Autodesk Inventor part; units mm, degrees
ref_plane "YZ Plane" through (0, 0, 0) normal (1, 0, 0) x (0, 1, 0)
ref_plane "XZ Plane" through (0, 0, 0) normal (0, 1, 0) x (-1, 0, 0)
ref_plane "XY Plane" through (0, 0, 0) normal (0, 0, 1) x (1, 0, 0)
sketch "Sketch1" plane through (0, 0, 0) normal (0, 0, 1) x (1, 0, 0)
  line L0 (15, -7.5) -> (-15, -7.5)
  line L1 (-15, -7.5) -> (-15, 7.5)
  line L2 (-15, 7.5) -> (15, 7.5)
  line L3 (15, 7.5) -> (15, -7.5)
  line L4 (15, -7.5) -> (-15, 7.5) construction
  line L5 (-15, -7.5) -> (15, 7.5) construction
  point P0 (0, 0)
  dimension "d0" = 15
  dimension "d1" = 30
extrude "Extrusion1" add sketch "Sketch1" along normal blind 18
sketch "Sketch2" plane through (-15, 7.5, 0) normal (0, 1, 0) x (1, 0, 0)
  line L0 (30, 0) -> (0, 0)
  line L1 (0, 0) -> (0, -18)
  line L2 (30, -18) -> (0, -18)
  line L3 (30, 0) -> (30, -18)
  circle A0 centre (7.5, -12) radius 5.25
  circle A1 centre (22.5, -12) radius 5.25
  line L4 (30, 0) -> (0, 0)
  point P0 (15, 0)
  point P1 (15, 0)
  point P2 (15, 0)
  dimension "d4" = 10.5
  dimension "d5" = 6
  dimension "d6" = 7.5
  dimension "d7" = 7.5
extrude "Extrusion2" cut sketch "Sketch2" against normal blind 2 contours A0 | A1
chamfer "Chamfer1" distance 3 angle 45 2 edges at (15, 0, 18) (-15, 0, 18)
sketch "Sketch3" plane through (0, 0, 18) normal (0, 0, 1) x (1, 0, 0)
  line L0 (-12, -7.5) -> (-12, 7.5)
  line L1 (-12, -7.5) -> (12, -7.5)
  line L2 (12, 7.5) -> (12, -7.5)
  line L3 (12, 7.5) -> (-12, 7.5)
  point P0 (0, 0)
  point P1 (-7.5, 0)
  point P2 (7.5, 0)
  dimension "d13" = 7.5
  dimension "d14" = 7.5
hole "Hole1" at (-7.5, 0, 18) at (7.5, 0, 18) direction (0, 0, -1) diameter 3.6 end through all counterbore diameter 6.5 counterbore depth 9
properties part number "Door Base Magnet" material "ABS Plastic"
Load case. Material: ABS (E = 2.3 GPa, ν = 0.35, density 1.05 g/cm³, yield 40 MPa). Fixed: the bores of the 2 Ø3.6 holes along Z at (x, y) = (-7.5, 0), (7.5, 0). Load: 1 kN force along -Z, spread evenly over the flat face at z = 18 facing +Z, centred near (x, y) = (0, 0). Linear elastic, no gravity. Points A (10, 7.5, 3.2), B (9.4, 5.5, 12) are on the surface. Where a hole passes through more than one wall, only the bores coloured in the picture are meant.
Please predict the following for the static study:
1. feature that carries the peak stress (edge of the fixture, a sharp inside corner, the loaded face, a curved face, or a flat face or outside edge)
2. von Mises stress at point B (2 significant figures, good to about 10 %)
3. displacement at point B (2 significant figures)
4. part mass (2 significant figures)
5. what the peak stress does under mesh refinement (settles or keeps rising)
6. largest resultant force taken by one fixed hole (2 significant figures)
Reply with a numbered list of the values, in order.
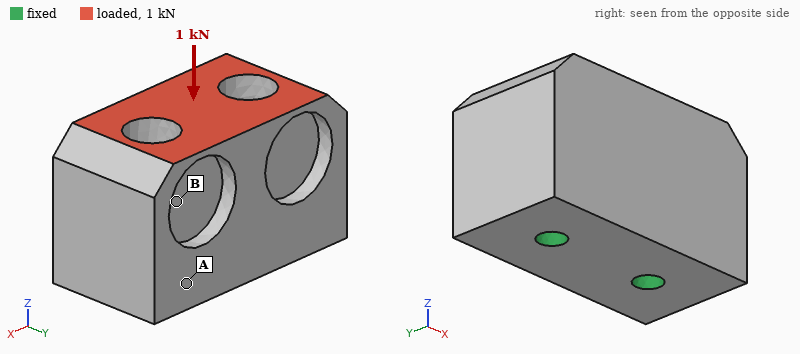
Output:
1. edge of the fixture
2. 5.4 MPa
3. 22 µm
4. 7.2 g
5. keeps rising
6. 510 N
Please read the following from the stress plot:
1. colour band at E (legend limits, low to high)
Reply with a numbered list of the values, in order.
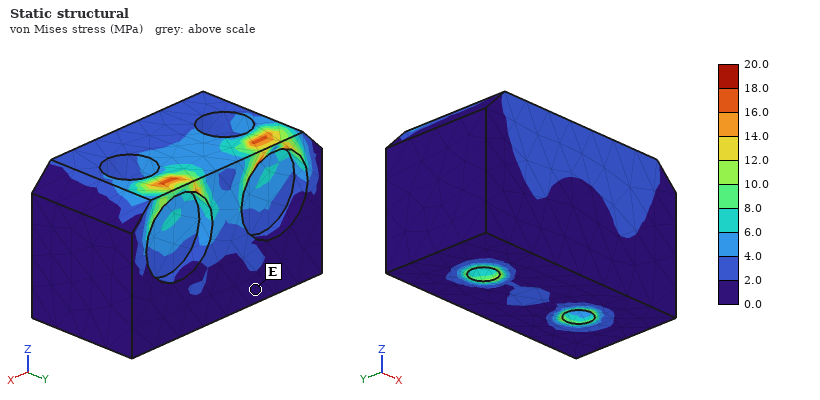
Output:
1. 0.0 to 2.0 MPa
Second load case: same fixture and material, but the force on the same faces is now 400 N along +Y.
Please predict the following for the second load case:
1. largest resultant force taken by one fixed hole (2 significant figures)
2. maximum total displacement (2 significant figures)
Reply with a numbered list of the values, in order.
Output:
1. 200 N
2. 0.13 mm
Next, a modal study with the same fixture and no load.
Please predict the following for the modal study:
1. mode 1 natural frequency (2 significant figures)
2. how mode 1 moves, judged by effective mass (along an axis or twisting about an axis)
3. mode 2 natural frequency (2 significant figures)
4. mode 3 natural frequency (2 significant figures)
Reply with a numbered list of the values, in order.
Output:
1. 7800 Hz
2. along Y
3. 11 kHz
4. 11 kHz
